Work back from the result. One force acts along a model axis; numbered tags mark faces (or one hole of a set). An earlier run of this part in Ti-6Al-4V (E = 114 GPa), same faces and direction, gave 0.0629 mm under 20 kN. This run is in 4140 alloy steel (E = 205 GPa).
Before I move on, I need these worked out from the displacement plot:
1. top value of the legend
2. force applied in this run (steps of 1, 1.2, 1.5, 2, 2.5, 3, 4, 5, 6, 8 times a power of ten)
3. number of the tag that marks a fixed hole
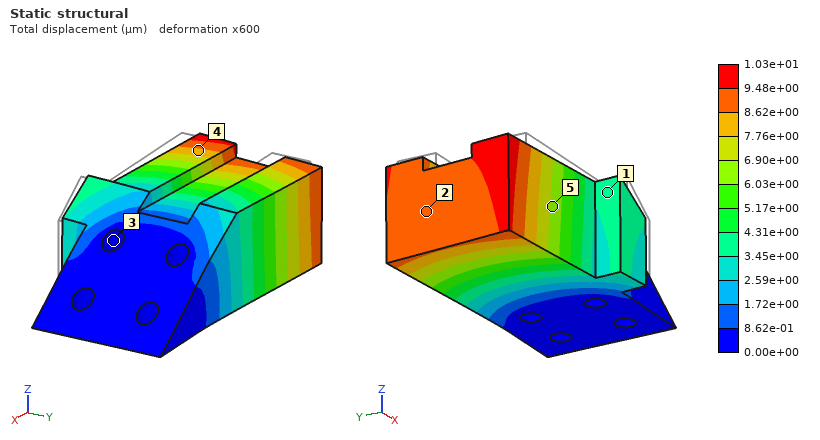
1.03e+01 µm
6 kN
3
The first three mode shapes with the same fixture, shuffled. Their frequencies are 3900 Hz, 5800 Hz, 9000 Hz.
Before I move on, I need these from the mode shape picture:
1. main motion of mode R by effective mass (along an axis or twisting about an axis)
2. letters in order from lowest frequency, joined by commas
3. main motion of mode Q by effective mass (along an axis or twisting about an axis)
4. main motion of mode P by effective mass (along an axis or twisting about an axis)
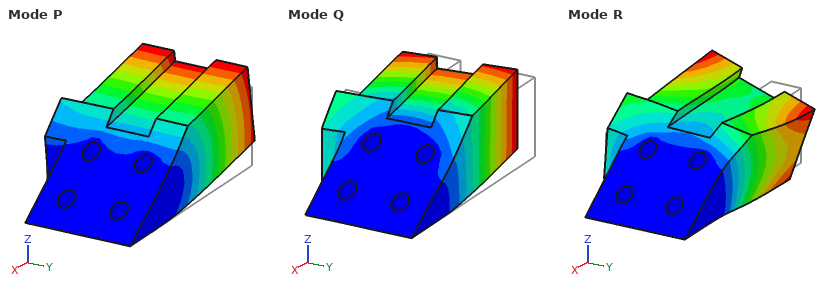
twisting about X
P, Q, R
along Y
along Z
